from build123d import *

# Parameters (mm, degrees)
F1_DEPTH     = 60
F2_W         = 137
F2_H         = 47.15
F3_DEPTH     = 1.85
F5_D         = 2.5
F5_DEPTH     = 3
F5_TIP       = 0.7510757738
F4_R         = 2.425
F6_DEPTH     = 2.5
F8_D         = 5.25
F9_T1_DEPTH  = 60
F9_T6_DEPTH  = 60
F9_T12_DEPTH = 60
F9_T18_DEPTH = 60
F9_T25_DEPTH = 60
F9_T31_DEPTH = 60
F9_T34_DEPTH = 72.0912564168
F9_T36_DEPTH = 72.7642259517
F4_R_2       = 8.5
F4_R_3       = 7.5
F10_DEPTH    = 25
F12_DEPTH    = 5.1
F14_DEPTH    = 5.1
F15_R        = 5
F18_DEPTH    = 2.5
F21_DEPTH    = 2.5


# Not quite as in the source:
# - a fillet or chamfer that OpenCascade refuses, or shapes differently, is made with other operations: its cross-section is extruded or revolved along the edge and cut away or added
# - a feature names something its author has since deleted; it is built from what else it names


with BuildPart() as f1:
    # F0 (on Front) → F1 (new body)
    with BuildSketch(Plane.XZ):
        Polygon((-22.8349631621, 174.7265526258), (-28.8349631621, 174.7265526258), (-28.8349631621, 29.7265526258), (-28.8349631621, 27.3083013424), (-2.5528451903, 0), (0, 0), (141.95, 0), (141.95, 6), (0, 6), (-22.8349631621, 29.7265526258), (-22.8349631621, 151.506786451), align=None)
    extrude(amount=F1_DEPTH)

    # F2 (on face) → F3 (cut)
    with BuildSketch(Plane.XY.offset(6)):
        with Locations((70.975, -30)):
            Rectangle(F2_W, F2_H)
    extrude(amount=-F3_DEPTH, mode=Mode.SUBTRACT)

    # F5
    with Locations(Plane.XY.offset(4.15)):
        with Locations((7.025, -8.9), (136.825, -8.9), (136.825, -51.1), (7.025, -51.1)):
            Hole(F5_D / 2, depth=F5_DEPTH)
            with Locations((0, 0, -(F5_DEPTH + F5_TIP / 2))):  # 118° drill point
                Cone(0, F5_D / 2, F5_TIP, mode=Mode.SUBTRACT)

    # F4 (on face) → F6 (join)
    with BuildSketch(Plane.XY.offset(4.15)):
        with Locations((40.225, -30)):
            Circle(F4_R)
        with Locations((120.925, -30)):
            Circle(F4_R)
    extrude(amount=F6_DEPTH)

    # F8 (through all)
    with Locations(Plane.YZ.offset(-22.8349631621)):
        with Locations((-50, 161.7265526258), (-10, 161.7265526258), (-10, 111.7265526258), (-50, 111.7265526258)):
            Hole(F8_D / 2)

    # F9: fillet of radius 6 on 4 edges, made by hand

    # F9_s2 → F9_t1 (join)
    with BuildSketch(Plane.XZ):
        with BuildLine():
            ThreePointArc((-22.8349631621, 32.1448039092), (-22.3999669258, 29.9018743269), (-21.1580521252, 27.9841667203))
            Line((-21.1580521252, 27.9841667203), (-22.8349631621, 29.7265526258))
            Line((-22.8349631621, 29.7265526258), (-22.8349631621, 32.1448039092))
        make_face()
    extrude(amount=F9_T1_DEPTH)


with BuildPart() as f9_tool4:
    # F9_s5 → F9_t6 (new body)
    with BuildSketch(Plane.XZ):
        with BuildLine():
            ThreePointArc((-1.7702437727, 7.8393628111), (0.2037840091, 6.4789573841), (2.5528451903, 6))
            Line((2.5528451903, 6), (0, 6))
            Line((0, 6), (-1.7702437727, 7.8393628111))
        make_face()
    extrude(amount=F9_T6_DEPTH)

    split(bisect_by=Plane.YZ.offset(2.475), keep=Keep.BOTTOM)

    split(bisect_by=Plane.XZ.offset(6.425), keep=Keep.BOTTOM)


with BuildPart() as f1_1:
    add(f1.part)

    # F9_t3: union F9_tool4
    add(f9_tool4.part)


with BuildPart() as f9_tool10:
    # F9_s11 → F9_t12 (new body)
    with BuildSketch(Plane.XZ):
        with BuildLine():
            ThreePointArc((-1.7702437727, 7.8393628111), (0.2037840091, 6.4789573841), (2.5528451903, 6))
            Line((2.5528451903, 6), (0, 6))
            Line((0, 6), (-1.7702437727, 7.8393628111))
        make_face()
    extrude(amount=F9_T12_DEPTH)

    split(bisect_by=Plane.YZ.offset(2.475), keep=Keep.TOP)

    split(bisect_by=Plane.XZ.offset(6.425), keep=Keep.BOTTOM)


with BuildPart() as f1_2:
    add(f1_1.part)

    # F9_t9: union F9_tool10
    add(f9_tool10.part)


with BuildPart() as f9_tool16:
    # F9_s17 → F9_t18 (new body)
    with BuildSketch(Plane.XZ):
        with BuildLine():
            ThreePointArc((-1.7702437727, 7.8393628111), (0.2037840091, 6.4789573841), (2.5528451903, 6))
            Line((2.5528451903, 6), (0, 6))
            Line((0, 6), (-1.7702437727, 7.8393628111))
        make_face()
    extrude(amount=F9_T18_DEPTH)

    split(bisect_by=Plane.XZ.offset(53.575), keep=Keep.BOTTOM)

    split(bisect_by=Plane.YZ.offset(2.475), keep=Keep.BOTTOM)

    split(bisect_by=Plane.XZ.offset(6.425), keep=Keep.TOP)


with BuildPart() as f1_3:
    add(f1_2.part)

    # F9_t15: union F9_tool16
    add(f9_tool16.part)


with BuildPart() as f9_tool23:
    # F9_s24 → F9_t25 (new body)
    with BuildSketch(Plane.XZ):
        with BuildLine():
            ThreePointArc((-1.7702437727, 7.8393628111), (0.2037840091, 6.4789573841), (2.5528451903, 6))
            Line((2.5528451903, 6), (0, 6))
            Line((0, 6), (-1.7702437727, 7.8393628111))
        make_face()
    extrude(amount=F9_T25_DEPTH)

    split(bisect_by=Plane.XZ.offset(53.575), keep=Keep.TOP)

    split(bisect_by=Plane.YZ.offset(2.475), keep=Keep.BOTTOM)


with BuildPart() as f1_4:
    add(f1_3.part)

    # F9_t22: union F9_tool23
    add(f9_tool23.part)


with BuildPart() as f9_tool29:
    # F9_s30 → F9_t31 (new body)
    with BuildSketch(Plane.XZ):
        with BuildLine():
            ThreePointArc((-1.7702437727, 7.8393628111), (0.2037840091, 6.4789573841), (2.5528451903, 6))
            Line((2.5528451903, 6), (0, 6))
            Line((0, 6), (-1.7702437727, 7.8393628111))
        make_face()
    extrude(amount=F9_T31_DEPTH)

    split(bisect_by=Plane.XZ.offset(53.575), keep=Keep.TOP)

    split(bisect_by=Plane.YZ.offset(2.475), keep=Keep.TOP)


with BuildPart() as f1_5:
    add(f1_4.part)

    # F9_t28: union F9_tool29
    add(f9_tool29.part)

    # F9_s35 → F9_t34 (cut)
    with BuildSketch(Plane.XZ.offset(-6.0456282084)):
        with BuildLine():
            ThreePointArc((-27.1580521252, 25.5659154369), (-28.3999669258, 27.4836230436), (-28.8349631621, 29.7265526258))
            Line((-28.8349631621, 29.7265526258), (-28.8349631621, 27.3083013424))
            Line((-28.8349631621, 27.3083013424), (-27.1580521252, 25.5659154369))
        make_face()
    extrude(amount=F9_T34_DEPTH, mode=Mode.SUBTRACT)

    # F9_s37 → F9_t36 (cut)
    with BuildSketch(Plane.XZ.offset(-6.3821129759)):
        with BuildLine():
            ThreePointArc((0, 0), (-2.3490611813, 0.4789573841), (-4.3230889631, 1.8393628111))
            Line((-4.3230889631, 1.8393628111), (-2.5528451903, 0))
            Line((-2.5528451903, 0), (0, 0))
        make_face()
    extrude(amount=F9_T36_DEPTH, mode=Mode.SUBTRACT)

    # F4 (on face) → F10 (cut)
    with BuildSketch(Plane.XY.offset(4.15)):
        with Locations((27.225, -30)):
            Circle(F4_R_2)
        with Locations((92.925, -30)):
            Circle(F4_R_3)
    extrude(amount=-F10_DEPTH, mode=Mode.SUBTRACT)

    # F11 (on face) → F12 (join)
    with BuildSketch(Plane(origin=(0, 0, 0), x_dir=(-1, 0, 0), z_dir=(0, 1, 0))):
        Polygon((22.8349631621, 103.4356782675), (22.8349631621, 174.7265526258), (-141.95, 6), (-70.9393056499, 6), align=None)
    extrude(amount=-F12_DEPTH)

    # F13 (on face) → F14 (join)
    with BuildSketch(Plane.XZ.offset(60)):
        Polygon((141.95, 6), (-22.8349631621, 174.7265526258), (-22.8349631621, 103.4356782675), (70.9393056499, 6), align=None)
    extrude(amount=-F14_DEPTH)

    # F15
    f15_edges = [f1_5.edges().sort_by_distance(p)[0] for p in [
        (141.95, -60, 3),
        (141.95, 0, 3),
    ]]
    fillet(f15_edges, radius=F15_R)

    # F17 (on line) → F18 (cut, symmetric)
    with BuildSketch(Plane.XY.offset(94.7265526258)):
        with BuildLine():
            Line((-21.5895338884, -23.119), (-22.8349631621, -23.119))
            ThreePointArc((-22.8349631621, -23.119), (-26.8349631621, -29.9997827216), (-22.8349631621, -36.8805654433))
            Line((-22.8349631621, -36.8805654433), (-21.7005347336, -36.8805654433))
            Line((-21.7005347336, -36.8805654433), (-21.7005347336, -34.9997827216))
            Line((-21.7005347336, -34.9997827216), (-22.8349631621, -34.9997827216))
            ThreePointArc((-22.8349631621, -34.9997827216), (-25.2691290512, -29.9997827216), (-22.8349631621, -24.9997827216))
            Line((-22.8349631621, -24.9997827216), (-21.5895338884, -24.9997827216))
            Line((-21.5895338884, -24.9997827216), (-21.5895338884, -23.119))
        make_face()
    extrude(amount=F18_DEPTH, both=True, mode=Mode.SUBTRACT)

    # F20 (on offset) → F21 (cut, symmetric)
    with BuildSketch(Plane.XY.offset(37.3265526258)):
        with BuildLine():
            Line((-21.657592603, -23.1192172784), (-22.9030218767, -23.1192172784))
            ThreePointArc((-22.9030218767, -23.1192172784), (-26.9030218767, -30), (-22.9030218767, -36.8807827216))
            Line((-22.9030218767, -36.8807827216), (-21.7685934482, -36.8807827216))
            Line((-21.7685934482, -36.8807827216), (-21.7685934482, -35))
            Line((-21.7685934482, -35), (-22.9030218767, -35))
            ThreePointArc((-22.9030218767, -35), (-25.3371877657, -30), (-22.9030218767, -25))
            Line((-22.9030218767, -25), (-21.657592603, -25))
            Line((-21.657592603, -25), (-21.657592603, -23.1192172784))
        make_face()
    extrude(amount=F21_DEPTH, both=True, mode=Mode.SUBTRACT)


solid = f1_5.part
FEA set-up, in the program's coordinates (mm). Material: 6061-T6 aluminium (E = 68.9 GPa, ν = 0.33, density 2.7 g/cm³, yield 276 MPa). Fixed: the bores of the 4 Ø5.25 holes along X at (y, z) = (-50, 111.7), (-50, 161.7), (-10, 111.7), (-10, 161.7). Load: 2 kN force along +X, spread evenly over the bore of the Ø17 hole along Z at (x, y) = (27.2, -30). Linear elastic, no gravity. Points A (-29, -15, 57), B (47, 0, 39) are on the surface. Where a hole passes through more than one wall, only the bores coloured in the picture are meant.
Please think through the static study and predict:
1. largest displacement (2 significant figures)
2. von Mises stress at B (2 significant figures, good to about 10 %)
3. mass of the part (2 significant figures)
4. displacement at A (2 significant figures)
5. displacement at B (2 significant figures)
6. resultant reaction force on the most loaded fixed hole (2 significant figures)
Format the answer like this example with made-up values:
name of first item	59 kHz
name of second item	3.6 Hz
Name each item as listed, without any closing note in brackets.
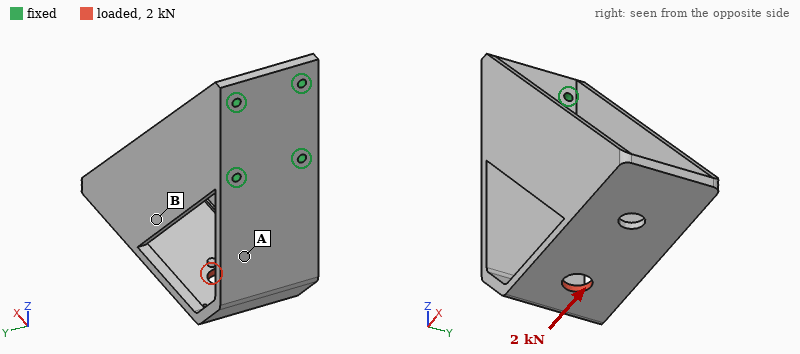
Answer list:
largest displacement	0.58 mm
von Mises stress at B	19 MPa
mass of the part	530 g
displacement at A	0.15 mm
displacement at B	0.25 mm
resultant reaction force on the most loaded fixed hole	3.2 kN
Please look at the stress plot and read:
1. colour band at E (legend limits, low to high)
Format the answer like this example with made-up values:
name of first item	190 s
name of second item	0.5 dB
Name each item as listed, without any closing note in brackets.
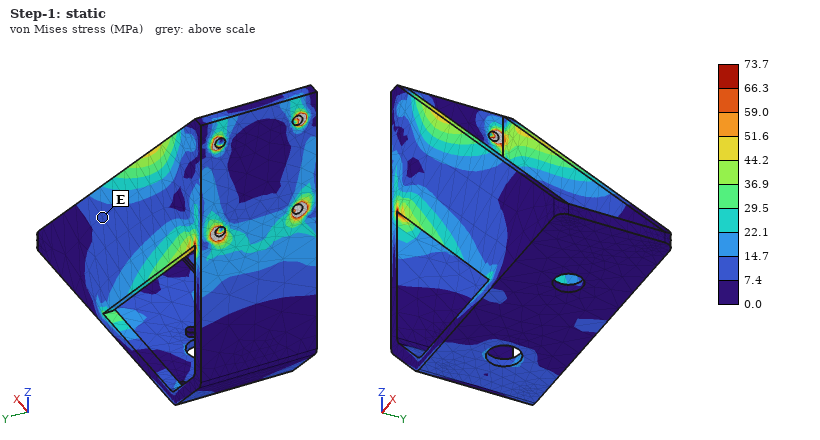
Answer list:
colour band at E	7.4 to 14.7 MPa
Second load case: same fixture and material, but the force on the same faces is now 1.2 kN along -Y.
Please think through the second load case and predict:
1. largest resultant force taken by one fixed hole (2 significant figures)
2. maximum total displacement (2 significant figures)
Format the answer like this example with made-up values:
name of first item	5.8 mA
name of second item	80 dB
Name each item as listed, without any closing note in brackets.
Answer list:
largest resultant force taken by one fixed hole	3.6 kN
maximum total displacement	1.3 mm
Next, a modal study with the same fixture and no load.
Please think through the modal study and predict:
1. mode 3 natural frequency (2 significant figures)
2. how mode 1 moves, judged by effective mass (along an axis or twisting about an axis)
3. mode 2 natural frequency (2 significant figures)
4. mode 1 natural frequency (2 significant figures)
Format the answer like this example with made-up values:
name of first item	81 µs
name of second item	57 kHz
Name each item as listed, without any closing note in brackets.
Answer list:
mode 3 natural frequency	740 Hz
how mode 1 moves, judged by effective mass	along Y
mode 2 natural frequency	660 Hz
mode 1 natural frequency	260 Hz
